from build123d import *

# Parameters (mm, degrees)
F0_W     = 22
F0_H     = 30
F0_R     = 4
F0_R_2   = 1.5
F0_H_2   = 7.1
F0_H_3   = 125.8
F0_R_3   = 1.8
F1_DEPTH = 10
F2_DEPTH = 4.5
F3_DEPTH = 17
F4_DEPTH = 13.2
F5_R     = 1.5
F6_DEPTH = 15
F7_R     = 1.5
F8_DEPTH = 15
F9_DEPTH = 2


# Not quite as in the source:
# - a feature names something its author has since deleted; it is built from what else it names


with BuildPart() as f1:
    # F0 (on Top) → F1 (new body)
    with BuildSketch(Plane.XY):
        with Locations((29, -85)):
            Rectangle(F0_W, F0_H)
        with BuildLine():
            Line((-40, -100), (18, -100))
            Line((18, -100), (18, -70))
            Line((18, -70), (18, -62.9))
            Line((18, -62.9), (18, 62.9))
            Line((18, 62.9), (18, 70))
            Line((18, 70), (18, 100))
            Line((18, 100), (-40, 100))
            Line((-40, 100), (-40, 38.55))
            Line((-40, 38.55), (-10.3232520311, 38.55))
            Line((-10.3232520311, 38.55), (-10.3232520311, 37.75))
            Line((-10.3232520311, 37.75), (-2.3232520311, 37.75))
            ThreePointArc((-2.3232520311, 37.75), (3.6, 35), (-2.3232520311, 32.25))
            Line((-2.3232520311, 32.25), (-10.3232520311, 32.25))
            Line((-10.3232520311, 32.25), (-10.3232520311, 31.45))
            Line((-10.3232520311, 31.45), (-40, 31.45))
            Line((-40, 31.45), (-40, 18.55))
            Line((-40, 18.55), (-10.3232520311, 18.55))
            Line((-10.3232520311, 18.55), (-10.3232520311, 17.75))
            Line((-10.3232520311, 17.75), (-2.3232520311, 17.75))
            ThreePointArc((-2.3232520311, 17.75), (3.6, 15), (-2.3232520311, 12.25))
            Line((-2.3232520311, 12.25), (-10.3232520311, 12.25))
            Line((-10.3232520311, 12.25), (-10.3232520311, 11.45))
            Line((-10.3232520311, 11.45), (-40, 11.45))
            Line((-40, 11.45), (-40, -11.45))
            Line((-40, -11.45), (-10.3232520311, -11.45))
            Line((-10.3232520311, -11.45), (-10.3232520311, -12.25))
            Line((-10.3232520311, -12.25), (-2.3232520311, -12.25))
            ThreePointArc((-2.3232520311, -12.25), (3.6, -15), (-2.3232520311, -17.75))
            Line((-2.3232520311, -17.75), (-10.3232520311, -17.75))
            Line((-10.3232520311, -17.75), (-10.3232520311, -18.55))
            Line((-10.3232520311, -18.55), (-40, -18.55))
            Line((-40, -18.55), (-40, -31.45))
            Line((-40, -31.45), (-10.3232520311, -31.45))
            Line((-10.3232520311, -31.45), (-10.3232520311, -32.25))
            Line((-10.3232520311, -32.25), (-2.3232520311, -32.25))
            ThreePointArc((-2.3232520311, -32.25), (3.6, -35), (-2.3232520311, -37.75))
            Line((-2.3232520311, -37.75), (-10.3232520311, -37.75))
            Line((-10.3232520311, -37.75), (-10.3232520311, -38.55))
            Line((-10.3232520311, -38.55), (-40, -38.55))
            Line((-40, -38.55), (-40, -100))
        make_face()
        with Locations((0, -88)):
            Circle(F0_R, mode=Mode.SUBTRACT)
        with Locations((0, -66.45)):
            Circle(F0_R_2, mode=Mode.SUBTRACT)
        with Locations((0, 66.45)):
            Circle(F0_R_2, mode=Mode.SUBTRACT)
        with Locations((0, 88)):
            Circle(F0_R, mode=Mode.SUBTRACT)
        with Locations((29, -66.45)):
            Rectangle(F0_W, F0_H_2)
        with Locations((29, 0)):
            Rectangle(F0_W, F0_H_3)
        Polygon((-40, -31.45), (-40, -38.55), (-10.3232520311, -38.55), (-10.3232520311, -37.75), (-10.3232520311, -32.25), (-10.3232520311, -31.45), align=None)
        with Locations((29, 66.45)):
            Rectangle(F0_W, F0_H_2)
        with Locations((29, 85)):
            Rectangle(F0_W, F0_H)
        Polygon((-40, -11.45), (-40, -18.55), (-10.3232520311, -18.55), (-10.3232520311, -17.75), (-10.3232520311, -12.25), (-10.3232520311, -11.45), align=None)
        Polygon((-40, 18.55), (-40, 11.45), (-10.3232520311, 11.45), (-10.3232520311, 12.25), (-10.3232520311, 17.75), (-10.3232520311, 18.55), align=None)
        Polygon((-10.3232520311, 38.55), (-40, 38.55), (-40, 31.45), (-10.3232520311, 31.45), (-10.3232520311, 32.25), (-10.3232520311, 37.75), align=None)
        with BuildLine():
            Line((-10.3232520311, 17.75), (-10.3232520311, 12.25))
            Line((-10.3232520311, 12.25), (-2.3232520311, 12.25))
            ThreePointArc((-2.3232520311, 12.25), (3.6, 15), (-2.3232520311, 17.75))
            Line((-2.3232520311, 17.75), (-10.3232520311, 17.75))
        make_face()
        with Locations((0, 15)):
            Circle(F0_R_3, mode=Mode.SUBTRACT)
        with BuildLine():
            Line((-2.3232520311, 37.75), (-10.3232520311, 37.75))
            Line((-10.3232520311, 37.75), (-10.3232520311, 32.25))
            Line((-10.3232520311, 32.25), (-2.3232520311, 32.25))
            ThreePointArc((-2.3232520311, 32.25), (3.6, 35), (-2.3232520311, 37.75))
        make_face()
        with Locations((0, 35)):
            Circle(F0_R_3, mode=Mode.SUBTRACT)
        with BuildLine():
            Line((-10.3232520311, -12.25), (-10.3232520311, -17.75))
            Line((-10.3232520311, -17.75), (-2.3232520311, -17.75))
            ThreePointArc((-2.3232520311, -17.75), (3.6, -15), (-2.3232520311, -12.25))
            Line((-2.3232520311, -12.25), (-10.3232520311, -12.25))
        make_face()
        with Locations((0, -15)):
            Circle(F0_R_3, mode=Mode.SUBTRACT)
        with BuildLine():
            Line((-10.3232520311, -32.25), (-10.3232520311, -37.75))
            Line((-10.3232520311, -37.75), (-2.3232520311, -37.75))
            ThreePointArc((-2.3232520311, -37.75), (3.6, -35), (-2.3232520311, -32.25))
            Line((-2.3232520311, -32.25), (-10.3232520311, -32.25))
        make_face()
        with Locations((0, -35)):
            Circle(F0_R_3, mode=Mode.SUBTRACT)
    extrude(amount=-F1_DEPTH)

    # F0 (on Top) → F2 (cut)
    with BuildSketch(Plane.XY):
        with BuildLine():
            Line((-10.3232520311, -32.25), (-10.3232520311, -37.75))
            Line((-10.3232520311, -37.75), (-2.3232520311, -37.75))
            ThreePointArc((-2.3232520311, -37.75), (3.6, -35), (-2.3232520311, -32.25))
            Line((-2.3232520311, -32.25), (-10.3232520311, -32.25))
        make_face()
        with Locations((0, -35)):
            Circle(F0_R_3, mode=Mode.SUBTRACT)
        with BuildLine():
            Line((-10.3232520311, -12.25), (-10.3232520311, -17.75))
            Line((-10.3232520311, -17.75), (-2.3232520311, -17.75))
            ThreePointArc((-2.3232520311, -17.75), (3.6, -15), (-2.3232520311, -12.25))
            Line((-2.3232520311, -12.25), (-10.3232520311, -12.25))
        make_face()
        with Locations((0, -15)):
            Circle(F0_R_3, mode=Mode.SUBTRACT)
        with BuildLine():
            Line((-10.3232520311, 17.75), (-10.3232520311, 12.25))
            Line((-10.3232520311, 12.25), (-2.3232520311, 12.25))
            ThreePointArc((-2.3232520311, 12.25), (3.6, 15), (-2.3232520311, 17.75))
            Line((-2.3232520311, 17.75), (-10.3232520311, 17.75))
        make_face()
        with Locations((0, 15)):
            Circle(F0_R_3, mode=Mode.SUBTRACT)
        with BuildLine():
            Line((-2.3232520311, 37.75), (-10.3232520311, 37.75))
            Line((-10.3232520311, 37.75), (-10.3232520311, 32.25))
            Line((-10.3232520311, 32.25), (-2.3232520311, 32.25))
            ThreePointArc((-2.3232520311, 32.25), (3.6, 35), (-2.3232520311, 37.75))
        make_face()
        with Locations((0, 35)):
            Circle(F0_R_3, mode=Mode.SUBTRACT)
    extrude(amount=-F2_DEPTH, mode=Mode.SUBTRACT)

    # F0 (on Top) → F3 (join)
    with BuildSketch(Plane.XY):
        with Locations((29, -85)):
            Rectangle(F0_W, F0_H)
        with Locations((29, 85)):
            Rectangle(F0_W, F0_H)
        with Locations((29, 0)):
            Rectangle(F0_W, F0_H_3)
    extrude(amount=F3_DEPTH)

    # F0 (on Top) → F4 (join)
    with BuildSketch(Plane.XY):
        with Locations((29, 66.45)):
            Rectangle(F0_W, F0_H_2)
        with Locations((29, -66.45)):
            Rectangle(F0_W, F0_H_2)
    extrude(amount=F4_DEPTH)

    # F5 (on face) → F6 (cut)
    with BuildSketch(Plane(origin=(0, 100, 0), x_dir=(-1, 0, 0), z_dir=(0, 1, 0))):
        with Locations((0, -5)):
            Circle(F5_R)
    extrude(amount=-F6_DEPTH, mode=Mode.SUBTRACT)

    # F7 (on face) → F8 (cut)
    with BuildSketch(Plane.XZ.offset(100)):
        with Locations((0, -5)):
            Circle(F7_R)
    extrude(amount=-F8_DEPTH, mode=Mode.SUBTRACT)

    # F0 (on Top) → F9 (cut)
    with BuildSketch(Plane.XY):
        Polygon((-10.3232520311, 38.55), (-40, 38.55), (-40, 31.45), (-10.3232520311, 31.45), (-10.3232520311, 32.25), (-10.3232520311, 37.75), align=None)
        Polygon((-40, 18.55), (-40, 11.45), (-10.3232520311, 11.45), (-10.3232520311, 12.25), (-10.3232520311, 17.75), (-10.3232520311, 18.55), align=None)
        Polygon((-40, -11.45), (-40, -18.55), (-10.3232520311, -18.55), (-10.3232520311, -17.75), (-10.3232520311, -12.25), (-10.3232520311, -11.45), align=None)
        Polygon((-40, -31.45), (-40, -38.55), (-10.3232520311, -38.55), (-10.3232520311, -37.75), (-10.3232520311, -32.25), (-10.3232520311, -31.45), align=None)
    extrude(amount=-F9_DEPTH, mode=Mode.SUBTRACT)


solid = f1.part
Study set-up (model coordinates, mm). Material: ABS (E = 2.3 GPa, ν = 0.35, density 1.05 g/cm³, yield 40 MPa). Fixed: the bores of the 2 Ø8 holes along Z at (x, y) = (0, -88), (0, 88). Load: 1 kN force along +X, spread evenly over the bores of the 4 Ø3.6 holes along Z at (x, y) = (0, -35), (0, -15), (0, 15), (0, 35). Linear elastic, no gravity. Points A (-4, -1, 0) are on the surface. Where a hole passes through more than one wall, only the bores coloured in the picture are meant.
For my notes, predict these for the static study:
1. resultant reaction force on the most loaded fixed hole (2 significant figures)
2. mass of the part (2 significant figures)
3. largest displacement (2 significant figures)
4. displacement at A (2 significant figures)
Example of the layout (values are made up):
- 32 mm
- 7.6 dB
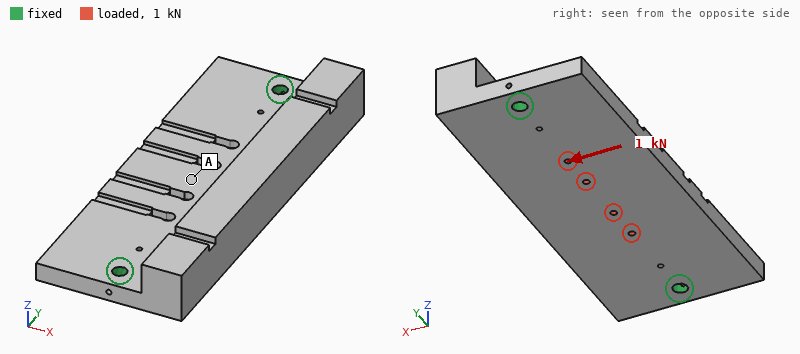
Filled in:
- 510 N
- 240 g
- 0.28 mm
- 0.19 mm
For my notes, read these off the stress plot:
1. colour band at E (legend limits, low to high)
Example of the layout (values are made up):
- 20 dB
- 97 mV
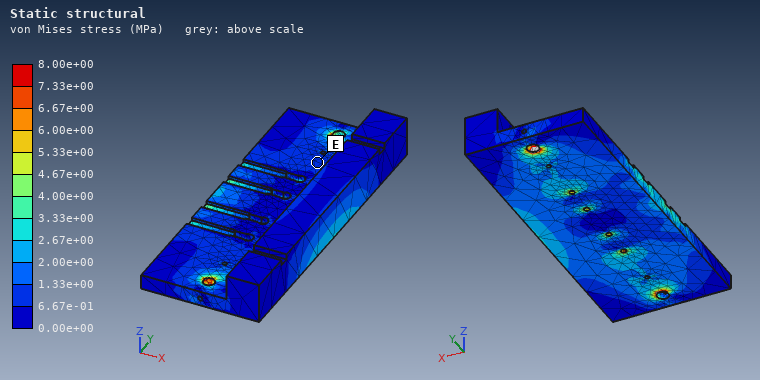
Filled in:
- 6.67e-01 to 1.33e+00 MPa
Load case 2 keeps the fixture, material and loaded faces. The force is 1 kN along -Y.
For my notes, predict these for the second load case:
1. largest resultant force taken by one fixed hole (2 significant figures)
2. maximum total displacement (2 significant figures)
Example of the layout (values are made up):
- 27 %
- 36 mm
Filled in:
- 500 N
- 48 µm
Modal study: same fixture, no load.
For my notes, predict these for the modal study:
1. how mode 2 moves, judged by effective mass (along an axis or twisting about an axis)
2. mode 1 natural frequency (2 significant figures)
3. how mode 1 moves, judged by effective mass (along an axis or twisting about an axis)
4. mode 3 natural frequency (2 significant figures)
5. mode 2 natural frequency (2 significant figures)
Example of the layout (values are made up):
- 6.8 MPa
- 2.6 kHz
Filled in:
- along Z
- 430 Hz
- along Z
- 1000 Hz
- 530 Hz
